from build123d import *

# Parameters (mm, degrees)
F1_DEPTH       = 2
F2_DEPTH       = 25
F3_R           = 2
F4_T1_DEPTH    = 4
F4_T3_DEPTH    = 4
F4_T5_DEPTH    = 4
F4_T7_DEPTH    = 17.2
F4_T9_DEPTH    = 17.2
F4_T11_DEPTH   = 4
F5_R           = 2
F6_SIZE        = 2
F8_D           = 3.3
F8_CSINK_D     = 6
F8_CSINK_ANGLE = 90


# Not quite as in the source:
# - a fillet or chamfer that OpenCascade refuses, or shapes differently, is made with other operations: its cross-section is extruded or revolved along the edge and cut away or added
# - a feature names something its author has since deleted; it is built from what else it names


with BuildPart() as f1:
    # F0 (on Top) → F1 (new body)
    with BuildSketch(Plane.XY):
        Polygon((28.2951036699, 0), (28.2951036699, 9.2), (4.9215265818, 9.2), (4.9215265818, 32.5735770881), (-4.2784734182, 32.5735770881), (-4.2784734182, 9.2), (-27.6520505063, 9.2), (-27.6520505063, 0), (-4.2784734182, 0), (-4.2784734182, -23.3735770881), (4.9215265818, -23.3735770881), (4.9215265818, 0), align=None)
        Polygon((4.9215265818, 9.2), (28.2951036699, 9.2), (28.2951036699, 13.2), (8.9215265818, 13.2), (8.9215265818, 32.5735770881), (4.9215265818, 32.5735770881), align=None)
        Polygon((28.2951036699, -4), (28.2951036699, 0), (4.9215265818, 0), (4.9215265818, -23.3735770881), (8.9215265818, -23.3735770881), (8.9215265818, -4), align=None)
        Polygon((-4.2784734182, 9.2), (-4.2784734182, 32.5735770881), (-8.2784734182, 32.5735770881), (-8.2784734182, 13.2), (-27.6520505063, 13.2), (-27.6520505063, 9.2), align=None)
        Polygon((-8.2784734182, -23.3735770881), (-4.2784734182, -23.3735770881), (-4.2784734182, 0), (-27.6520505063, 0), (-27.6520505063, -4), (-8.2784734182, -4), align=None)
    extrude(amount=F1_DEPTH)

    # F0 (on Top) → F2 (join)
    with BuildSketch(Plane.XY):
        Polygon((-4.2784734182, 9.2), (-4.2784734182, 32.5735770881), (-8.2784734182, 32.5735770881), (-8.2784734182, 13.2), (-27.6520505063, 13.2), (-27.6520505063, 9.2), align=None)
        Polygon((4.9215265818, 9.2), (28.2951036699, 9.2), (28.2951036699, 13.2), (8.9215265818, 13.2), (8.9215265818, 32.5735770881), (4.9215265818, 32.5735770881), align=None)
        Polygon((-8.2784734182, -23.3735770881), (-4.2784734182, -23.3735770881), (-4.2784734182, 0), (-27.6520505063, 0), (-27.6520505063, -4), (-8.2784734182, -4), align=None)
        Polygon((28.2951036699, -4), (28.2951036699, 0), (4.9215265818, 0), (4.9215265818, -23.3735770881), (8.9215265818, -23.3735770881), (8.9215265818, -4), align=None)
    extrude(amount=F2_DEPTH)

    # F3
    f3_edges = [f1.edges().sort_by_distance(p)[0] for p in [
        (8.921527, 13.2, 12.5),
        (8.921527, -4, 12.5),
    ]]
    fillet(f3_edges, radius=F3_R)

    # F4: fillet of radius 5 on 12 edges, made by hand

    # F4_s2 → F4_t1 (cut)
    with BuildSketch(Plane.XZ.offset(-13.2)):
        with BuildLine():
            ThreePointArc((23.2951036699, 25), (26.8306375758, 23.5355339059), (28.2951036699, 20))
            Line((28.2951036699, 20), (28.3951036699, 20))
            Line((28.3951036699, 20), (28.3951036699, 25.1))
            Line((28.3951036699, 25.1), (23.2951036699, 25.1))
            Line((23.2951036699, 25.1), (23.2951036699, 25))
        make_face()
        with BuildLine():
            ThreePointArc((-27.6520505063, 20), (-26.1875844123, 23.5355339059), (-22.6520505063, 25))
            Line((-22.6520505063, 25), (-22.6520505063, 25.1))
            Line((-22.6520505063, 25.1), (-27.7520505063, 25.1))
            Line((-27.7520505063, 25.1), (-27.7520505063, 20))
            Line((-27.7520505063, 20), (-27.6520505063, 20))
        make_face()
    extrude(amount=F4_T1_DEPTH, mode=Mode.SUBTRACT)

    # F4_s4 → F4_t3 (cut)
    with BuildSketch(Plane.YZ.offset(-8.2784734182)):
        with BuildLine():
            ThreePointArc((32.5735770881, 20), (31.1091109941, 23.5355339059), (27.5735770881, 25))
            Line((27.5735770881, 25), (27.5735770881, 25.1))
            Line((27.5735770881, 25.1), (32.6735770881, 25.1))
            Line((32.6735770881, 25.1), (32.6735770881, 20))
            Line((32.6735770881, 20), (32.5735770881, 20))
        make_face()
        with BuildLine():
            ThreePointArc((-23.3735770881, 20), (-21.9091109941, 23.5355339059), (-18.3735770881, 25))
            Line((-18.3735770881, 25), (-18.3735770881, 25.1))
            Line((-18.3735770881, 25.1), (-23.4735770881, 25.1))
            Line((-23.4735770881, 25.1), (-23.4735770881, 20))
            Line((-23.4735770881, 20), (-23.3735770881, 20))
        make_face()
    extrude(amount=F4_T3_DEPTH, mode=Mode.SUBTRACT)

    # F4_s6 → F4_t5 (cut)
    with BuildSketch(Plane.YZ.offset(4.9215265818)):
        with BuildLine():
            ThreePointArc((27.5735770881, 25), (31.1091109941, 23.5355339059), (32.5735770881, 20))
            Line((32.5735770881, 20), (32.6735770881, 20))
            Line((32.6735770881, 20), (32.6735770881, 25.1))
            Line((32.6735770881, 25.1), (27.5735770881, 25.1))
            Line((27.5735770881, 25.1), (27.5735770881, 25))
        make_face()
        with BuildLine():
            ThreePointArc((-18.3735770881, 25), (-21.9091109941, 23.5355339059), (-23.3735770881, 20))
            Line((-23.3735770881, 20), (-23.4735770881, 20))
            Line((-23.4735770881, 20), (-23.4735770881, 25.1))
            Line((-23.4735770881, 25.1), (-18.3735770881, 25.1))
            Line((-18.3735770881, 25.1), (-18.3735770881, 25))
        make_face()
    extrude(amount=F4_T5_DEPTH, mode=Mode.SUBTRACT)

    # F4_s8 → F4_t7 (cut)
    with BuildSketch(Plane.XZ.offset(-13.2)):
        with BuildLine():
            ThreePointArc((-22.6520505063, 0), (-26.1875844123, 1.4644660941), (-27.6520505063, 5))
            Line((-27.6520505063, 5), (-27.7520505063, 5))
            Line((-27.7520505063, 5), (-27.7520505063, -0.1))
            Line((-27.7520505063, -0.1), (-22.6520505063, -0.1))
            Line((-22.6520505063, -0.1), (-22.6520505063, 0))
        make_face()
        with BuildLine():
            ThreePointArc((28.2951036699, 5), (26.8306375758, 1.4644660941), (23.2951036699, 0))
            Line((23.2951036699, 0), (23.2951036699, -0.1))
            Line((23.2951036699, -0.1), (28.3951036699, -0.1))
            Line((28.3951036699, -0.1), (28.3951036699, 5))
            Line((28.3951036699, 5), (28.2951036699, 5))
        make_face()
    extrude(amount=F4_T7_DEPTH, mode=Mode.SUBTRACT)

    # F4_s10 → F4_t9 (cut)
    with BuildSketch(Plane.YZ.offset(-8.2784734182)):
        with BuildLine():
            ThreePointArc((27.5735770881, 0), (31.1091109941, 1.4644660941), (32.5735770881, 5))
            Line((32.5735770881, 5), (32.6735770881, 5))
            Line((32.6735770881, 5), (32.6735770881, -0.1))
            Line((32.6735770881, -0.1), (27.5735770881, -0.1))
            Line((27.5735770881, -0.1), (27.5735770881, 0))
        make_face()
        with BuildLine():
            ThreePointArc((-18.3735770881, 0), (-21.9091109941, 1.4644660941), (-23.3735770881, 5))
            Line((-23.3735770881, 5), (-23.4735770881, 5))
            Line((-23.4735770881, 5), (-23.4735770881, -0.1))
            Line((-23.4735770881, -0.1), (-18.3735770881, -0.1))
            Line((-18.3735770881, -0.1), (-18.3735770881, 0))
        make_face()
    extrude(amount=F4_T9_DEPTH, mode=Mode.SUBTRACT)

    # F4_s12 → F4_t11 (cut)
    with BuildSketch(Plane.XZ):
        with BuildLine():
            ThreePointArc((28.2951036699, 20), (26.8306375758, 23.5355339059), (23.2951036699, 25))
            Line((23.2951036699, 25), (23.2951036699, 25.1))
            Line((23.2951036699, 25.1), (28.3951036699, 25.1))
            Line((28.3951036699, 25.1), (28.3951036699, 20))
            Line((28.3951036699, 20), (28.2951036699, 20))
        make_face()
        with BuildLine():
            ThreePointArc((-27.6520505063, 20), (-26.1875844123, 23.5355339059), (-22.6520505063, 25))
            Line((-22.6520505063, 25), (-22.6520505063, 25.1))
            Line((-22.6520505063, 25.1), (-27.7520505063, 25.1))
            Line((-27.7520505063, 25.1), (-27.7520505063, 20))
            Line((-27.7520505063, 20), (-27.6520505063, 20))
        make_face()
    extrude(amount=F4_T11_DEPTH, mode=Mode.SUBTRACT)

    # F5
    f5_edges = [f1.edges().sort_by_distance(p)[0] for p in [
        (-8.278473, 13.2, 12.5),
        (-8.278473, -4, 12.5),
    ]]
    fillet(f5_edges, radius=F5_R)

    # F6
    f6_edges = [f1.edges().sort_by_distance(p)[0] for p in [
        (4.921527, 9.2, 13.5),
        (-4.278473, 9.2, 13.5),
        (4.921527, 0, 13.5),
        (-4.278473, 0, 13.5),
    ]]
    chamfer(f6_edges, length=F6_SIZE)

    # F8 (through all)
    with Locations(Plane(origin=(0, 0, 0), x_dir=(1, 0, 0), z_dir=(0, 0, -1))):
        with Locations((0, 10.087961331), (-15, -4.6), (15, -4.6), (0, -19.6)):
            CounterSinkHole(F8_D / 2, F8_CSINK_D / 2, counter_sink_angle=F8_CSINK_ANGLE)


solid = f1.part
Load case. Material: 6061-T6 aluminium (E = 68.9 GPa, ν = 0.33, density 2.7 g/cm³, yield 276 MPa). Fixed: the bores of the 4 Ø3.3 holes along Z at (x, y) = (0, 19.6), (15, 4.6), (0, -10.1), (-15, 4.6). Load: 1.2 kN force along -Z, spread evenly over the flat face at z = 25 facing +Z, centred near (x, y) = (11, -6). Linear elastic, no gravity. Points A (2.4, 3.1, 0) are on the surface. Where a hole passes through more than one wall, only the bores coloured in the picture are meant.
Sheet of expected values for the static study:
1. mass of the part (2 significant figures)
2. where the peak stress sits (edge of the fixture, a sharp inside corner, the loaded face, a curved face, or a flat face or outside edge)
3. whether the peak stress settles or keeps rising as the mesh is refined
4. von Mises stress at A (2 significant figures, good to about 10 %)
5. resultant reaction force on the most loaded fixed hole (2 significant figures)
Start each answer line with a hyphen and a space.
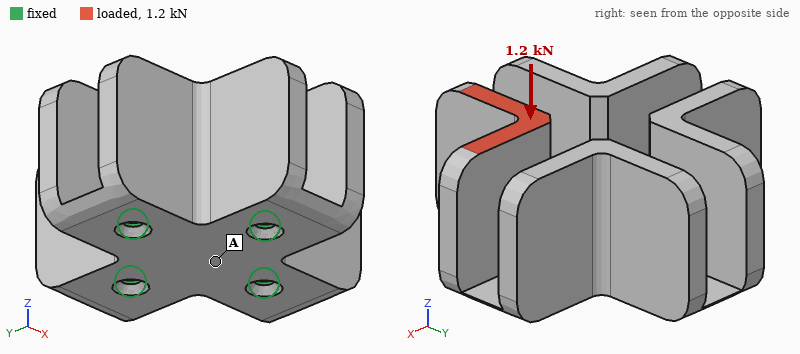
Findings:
- 49 g
- edge of the fixture
- keeps rising
- 34 MPa
- 720 N
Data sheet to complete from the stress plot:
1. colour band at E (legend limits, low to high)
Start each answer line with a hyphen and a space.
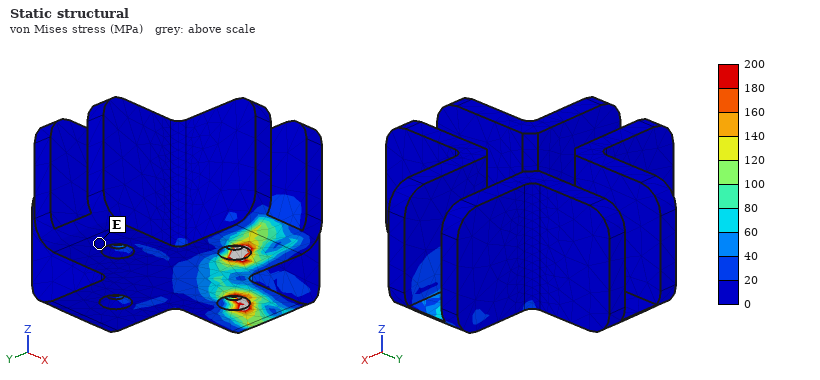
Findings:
- 0 to 20 MPa
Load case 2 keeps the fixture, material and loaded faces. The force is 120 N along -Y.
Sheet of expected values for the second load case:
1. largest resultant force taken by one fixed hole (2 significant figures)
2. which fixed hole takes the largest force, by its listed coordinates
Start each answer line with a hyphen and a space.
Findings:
- 210 N
- (0, -10.1)
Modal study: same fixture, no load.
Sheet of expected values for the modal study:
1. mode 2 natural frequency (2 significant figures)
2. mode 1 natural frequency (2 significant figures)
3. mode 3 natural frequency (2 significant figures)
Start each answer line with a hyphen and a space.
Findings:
- 2500 Hz
- 1900 Hz
- 2500 Hz
